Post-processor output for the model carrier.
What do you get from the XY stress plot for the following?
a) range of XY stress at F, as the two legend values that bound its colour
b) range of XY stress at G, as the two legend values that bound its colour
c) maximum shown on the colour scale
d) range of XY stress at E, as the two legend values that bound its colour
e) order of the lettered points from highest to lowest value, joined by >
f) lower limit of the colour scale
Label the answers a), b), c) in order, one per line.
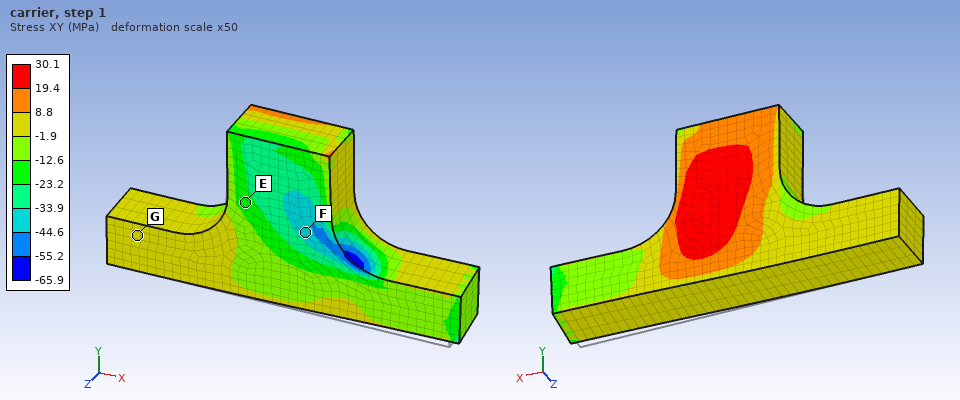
a) -44.6 to -33.9 MPa
b) -1.9 to 8.8 MPa
c) 30.1 MPa
d) -23.2 to -12.6 MPa
e) G > E > F
f) -65.9 MPa
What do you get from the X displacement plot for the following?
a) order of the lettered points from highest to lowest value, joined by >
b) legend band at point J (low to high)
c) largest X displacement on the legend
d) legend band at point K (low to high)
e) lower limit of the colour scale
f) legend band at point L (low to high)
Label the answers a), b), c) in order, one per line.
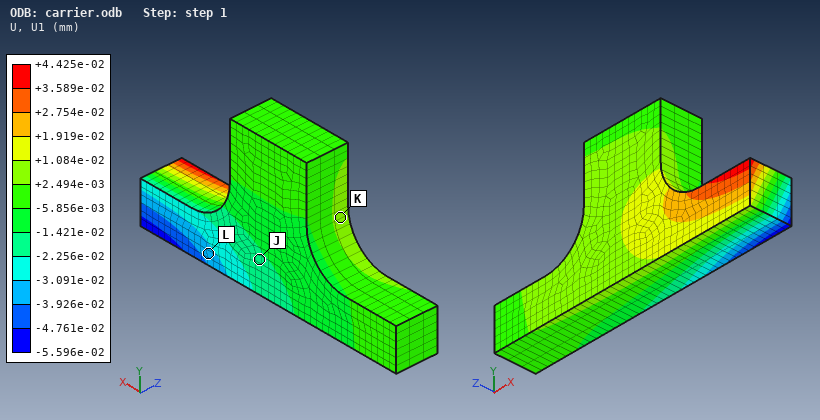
a) K > J > L
b) -2.256e-02 to -1.421e-02 mm
c) +4.425e-02 mm
d) +2.494e-03 to +1.084e-02 mm
e) -5.596e-02 mm
f) -3.926e-02 to -3.091e-02 mm
